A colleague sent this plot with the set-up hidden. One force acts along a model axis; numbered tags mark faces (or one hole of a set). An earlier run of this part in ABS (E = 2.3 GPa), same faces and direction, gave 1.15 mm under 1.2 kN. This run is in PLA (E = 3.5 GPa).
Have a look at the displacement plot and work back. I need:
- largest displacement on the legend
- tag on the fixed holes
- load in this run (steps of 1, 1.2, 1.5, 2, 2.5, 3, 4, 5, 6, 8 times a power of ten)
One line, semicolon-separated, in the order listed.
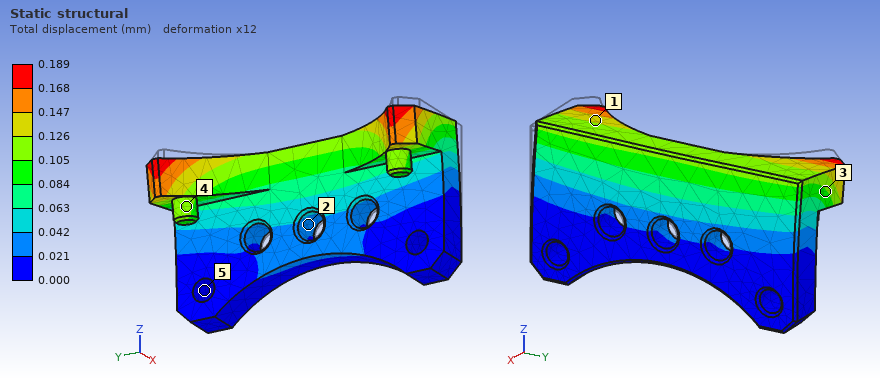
0.189 mm; 5; 300 N
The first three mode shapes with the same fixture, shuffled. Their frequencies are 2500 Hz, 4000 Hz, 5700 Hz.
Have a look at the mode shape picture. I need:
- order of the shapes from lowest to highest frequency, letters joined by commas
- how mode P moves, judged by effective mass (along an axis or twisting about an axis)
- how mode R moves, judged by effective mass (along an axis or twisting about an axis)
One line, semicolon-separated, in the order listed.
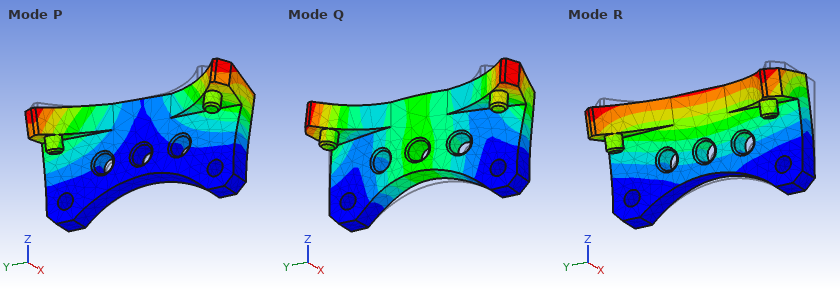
R, P, Q; twisting about Z; along X
